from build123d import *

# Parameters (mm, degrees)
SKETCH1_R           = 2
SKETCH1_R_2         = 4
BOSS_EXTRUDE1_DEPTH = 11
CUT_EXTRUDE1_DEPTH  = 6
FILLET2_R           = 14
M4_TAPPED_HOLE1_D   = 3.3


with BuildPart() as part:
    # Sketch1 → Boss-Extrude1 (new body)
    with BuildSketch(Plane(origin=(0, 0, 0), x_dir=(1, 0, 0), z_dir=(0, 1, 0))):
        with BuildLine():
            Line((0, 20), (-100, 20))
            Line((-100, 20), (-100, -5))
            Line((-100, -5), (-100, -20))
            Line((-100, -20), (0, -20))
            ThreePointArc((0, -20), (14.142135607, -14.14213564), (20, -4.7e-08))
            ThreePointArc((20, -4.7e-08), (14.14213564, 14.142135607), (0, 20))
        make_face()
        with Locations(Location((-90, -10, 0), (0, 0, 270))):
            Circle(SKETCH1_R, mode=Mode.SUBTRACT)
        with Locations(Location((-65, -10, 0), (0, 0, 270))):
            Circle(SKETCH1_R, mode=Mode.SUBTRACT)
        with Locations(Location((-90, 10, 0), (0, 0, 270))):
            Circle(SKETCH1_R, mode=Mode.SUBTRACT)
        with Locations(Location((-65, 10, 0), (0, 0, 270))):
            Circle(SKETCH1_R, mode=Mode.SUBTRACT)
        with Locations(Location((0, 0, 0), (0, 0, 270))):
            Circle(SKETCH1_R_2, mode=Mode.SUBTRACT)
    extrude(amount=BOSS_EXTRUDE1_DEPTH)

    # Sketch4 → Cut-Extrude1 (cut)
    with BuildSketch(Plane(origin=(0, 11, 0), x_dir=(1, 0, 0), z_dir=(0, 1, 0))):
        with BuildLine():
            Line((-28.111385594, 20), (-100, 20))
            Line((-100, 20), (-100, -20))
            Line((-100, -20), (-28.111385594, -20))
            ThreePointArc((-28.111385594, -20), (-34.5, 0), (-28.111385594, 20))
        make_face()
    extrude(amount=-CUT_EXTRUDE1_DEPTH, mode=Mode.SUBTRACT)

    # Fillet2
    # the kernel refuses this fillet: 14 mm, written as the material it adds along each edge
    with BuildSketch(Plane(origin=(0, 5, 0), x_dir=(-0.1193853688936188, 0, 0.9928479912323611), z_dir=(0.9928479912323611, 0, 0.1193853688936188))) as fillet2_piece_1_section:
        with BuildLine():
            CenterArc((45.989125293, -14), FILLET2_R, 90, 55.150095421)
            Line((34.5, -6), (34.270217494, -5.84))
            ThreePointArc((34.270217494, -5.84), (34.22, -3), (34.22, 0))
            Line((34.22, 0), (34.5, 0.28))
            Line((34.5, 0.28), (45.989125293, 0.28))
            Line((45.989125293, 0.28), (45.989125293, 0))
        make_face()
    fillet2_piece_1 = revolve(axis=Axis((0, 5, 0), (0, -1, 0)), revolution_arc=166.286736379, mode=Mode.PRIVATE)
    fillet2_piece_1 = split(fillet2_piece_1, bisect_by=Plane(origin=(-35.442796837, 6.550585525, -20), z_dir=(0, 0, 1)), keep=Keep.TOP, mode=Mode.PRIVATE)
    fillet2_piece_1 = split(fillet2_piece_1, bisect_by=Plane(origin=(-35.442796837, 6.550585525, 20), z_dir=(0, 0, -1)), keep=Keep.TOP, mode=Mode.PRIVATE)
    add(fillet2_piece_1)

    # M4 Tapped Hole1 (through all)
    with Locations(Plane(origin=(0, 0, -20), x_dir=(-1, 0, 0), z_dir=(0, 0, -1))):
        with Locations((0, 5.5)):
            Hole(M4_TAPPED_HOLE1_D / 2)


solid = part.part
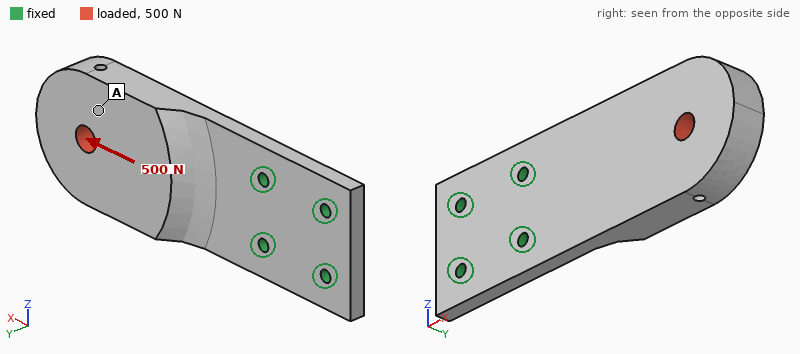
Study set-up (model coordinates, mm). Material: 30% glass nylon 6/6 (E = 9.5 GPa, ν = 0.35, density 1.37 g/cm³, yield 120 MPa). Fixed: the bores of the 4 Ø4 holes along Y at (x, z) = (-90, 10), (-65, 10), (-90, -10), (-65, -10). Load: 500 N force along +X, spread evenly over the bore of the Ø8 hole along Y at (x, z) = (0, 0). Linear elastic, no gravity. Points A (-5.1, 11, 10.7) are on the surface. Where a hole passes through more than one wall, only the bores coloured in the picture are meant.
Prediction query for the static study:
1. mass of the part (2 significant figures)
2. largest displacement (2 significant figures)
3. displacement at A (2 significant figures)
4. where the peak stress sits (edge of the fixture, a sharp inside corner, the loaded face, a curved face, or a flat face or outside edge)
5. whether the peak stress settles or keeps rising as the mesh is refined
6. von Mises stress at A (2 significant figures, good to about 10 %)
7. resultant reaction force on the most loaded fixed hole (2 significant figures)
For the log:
47 g
0.68 mm
0.45 mm
edge of the fixture
keeps rising
1.2 MPa
220 N
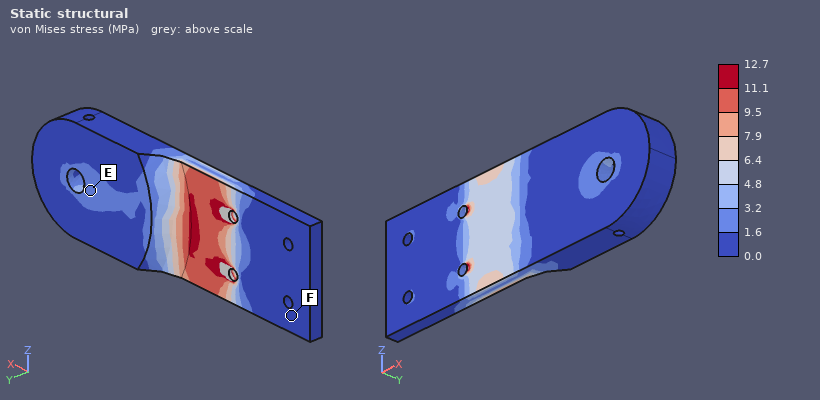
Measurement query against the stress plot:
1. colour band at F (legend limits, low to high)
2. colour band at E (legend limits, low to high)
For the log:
0.0 to 1.6 MPa
1.6 to 3.2 MPa
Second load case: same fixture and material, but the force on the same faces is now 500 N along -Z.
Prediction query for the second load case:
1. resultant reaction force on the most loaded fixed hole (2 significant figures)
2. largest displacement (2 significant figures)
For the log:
1.1 kN
0.35 mm
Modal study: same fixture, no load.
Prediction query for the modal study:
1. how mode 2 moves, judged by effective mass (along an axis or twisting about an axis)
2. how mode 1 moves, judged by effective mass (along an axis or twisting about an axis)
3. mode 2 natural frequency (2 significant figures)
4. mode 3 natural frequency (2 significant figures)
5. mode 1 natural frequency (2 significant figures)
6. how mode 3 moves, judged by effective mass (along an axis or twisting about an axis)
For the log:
along Z
along Y
1400 Hz
1500 Hz
250 Hz
along Z
